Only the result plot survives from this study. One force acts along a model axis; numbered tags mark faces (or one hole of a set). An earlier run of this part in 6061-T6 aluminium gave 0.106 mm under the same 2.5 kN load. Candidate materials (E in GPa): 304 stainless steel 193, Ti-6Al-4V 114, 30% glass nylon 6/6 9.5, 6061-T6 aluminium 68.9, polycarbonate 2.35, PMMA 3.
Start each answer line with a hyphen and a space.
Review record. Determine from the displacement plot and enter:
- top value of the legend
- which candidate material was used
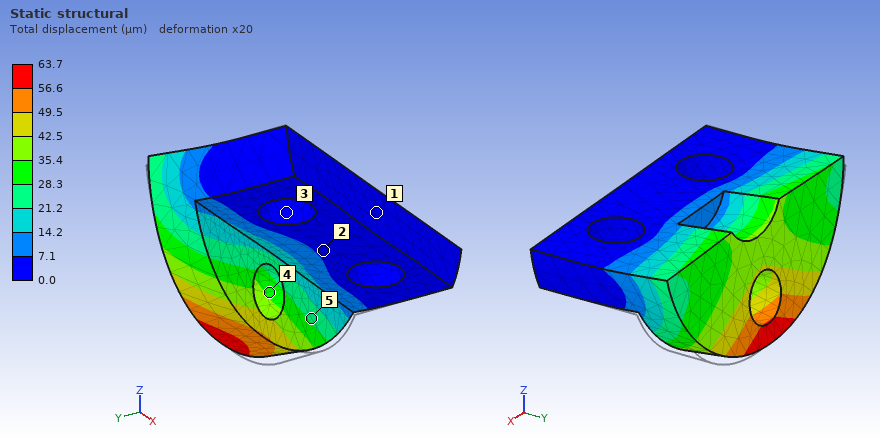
- 63.7 µm
- Ti-6Al-4V
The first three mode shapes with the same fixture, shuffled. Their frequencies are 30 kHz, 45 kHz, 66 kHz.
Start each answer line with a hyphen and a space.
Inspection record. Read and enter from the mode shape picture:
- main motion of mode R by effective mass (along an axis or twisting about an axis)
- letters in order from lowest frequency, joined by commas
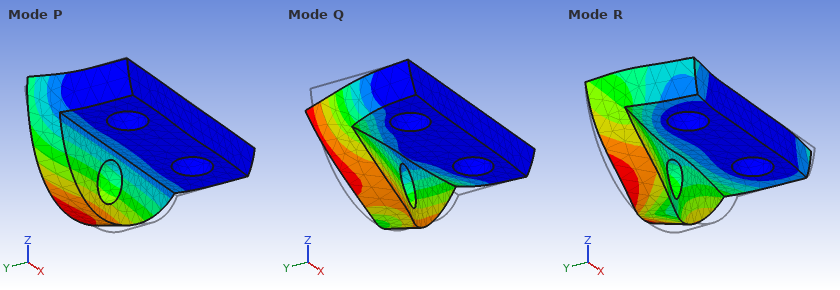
- along X
- P, Q, R
